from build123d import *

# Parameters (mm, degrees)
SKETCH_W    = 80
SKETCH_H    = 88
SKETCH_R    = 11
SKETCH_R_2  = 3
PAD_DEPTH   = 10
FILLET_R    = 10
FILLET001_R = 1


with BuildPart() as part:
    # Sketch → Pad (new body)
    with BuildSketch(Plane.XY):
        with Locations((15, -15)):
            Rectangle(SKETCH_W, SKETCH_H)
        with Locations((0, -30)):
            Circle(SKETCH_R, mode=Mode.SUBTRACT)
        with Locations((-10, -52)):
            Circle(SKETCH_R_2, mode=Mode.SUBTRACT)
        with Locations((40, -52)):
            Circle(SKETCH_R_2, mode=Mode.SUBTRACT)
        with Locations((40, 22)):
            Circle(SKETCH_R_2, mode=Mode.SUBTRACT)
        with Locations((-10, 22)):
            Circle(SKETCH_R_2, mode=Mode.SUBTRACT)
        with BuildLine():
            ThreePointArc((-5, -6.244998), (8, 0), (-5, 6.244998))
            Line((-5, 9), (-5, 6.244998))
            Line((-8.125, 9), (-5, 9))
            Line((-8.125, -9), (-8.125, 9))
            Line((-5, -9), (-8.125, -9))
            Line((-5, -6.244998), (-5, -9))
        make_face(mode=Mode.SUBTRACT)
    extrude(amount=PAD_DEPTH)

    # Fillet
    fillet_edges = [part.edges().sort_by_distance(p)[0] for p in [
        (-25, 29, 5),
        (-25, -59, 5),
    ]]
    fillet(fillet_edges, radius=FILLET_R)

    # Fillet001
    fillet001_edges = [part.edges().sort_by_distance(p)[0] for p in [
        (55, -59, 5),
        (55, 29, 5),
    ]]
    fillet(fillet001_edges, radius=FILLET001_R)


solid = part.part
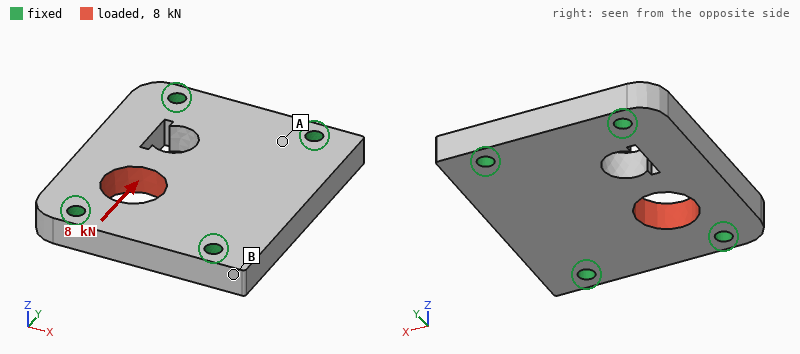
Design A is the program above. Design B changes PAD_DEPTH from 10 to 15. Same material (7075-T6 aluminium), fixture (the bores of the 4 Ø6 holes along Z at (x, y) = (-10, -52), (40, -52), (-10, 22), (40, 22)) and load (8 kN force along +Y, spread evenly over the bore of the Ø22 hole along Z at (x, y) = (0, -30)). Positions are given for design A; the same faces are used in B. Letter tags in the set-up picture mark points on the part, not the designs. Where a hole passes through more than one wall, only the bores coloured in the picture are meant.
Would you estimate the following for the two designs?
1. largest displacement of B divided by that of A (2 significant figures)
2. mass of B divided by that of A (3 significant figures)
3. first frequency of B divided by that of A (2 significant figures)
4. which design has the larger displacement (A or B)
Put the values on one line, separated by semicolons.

0.67; 1.50; 1.3; A
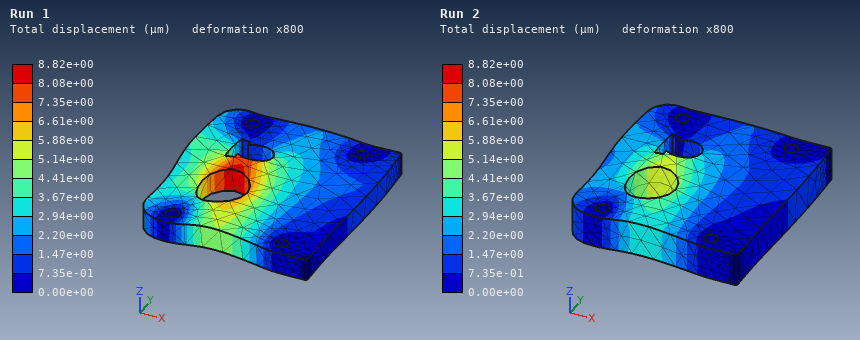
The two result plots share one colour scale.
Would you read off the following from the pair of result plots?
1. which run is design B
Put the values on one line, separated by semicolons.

Run 2
